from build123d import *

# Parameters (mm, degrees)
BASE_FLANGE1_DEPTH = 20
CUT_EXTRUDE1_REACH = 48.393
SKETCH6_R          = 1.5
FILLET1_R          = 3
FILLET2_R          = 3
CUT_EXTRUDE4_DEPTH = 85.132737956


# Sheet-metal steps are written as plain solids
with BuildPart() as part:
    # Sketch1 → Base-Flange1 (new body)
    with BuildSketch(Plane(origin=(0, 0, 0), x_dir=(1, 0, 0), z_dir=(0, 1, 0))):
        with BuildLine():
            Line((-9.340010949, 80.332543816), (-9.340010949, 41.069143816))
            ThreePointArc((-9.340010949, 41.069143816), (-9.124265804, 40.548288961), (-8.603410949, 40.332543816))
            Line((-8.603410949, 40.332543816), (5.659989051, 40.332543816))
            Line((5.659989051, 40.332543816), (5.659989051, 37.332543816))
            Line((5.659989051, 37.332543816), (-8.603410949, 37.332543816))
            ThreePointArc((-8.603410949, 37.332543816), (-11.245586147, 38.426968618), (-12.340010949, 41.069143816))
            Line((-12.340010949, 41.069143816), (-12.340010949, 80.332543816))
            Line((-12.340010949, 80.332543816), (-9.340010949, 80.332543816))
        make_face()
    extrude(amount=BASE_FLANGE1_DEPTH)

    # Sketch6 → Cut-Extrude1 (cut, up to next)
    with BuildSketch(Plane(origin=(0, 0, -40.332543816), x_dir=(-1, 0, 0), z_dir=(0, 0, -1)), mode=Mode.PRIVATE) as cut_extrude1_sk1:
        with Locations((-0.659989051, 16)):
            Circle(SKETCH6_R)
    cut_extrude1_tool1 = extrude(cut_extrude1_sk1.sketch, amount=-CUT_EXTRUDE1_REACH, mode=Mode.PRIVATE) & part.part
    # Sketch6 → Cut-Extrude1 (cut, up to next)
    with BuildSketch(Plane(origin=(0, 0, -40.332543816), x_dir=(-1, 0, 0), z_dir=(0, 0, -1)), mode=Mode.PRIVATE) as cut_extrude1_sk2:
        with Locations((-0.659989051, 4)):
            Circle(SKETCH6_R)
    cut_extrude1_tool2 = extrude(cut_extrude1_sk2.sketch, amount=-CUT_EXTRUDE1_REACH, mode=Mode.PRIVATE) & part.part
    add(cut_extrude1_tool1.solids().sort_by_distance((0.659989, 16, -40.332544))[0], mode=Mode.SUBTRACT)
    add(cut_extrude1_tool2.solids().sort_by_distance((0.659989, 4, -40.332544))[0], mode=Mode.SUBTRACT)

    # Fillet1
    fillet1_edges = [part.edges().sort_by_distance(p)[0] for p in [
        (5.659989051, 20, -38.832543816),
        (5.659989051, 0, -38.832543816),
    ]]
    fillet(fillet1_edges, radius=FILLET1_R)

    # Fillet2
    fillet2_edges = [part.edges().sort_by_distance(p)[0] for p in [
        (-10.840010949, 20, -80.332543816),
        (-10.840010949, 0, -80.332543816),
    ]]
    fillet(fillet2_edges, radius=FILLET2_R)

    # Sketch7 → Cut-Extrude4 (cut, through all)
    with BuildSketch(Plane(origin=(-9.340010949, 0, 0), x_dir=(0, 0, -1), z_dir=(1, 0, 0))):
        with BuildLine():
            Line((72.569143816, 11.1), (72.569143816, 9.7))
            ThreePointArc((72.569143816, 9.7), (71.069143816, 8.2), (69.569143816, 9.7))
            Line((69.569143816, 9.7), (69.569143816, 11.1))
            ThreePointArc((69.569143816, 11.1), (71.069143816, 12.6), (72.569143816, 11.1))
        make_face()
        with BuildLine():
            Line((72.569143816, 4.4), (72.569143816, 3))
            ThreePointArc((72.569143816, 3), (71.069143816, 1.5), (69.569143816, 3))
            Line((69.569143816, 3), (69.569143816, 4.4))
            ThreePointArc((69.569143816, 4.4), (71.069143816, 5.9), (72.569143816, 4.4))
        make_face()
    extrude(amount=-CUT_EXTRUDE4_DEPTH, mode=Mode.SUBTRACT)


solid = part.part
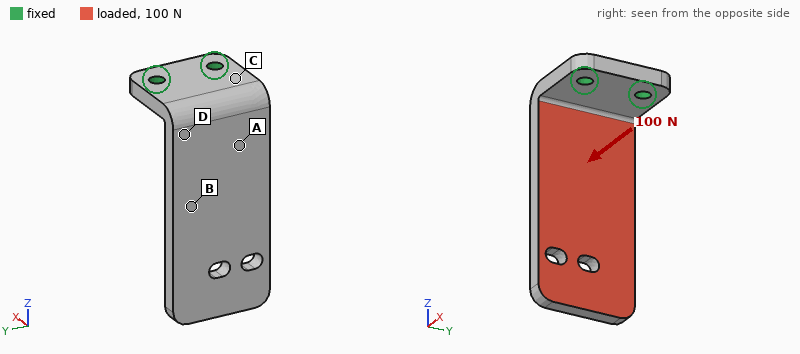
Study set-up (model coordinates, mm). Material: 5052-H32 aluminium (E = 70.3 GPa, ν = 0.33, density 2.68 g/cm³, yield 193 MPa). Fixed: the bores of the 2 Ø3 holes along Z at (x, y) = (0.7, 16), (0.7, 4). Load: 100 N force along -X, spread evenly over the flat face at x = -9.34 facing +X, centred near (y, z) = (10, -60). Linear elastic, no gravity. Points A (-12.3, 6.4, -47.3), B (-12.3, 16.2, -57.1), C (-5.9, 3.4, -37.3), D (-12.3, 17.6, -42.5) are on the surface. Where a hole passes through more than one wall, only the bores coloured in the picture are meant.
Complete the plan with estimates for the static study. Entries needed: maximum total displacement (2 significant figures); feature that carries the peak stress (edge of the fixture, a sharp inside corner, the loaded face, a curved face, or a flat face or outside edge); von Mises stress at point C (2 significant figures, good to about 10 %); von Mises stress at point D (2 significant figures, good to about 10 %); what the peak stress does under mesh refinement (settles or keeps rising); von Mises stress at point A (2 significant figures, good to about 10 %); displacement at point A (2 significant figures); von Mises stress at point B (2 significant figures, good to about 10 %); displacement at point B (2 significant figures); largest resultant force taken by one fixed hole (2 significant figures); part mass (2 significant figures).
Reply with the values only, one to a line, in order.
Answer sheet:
0.55 mm
edge of the fixture
65 MPa
57 MPa
keeps rising
41 MPa
0.094 mm
22 MPa
0.21 mm
57 N
8.8 g
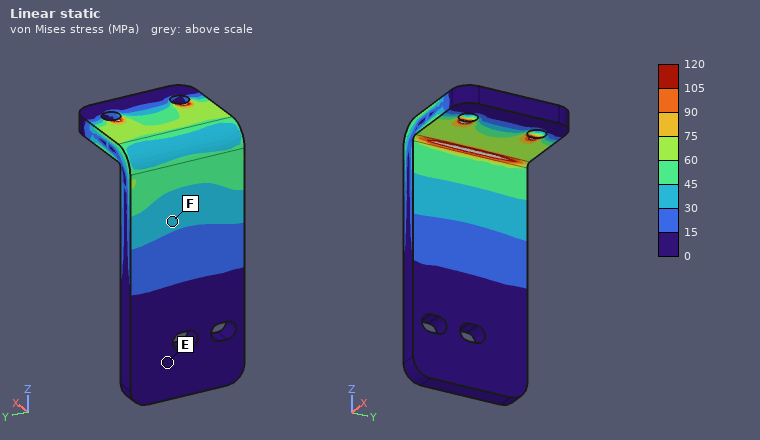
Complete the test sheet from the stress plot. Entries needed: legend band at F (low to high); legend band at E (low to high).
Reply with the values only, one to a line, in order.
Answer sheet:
30 to 45 MPa
0 to 15 MPa
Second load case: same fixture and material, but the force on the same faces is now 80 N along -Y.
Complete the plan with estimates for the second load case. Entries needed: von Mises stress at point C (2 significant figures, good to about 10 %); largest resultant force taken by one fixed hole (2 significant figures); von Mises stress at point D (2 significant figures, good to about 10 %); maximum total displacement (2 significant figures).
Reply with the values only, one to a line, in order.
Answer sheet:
26 MPa
140 N
14 MPa
92 µm
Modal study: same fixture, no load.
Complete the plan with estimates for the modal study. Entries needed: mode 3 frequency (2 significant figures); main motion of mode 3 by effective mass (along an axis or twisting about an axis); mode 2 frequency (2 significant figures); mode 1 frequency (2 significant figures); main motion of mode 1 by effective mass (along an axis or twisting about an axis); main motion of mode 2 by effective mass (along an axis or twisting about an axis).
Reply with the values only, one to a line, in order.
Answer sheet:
5600 Hz
along Z
2300 Hz
1100 Hz
along X
along Y
